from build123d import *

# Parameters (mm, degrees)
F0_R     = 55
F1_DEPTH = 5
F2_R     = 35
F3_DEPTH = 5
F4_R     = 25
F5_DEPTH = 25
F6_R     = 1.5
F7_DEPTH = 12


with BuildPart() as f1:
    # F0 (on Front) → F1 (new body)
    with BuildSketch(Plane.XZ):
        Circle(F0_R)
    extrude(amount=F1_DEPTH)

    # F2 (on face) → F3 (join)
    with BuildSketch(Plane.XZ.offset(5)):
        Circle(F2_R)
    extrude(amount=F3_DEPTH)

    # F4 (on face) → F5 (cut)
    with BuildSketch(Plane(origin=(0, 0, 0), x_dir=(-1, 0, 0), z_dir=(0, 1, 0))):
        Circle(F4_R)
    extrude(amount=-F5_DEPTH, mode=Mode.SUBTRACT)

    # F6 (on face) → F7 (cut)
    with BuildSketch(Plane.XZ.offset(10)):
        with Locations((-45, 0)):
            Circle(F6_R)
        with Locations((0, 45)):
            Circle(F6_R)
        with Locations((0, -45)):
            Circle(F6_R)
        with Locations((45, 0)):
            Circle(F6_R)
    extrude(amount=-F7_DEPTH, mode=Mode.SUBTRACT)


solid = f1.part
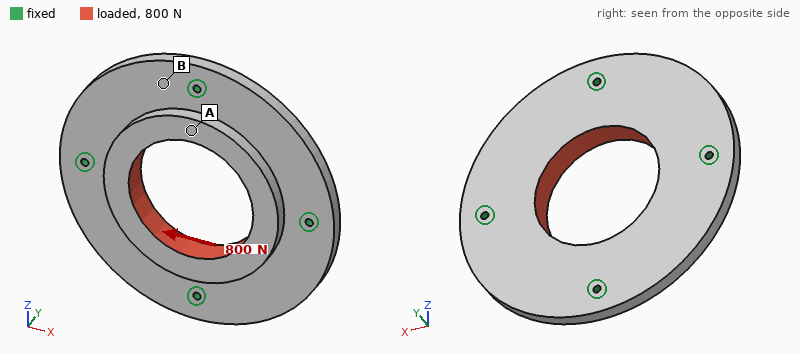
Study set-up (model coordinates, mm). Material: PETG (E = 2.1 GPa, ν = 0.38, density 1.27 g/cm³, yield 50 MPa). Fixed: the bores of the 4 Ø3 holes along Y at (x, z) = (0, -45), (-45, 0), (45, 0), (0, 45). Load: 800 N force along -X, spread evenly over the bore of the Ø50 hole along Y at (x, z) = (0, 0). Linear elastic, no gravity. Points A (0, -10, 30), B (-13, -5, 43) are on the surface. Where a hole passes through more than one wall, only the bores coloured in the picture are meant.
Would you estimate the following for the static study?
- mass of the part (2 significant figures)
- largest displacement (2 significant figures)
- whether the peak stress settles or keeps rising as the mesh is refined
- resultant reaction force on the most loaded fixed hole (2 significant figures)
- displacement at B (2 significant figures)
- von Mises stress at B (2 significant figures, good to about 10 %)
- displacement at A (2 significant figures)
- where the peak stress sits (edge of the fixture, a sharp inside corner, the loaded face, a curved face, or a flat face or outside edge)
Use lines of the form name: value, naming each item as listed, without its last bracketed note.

mass of the part: 60 g
largest displacement: 37 µm
whether the peak stress settles or keeps rising as the mesh is refined: keeps rising
resultant reaction force on the most loaded fixed hole: 210 N
displacement at B: 16 µm
von Mises stress at B: 1.1 MPa
displacement at A: 26 µm
where the peak stress sits: edge of the fixture
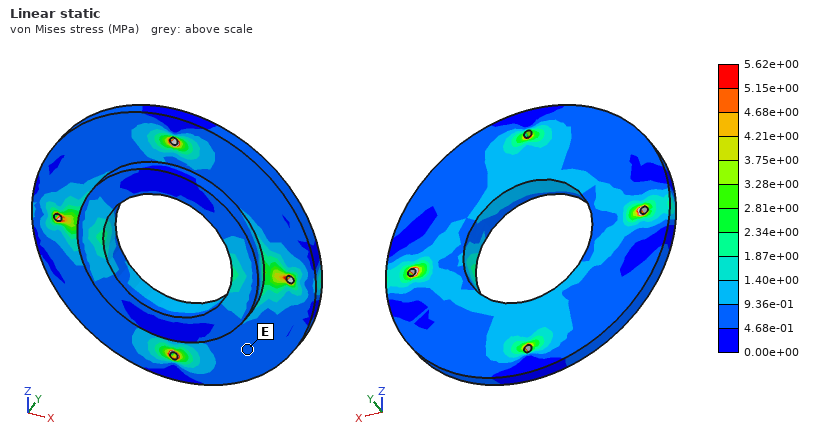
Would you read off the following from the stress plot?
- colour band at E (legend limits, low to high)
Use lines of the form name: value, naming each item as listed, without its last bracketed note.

colour band at E: 4.68e-01 to 9.36e-01 MPa
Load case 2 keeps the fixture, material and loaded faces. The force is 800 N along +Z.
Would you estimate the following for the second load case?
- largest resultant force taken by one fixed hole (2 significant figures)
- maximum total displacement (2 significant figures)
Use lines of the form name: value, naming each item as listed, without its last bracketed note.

largest resultant force taken by one fixed hole: 210 N
maximum total displacement: 37 µm
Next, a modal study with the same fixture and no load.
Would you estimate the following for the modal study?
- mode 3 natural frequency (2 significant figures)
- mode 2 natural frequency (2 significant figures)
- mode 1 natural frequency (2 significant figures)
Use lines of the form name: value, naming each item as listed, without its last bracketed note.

mode 3 natural frequency: 1300 Hz
mode 2 natural frequency: 1300 Hz
mode 1 natural frequency: 1100 Hz
